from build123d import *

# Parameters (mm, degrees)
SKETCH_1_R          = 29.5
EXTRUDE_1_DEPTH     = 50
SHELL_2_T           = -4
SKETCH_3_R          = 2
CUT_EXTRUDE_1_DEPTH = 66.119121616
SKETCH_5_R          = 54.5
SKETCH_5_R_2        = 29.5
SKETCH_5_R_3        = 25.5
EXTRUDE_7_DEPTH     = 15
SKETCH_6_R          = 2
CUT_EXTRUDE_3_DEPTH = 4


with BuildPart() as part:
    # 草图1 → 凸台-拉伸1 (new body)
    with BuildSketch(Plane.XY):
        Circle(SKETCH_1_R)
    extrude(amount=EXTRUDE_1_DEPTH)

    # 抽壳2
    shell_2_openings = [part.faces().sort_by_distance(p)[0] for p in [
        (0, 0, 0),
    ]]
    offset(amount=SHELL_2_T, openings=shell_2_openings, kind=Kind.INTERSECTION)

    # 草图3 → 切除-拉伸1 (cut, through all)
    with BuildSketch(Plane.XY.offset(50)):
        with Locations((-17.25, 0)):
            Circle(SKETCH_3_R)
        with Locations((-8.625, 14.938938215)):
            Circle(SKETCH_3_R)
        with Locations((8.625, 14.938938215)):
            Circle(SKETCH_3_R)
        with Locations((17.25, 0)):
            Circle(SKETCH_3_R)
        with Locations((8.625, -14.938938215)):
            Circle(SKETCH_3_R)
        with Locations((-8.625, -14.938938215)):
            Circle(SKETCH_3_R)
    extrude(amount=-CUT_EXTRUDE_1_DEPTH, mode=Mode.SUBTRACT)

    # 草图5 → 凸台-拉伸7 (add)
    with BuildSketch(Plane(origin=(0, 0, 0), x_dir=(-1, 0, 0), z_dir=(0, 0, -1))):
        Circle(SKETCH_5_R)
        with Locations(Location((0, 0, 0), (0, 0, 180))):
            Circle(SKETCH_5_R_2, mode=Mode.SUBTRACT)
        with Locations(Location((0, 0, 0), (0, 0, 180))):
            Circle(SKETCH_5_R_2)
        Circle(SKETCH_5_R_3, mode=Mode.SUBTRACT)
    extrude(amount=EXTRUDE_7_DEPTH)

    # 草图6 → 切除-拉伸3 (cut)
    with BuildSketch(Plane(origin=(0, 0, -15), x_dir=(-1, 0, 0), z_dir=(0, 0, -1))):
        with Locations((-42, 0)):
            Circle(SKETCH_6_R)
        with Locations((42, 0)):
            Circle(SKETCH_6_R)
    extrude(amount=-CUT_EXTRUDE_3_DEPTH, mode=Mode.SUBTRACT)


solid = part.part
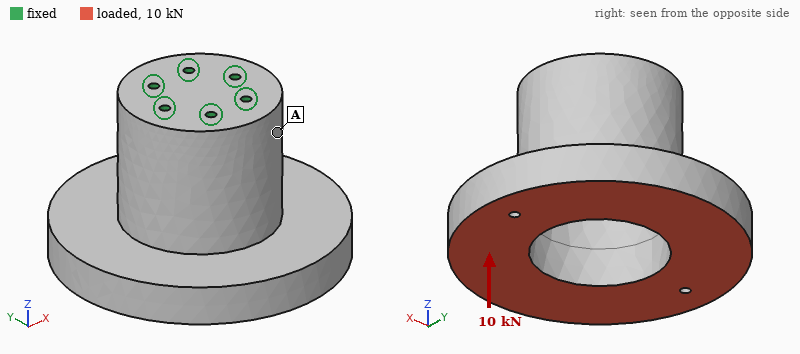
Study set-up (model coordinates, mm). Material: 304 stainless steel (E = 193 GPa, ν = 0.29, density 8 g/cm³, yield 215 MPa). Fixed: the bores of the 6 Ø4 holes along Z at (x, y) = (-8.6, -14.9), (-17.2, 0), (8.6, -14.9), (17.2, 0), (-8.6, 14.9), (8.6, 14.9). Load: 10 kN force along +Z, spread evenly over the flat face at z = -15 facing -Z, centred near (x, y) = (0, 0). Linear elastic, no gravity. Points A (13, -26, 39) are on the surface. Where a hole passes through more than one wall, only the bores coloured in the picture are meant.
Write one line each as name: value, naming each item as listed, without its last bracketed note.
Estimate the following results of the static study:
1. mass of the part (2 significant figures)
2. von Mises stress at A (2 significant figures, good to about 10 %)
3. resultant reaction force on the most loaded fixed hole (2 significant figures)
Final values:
mass of the part: 1.2 kg
von Mises stress at A: 20 MPa
resultant reaction force on the most loaded fixed hole: 1.7 kN
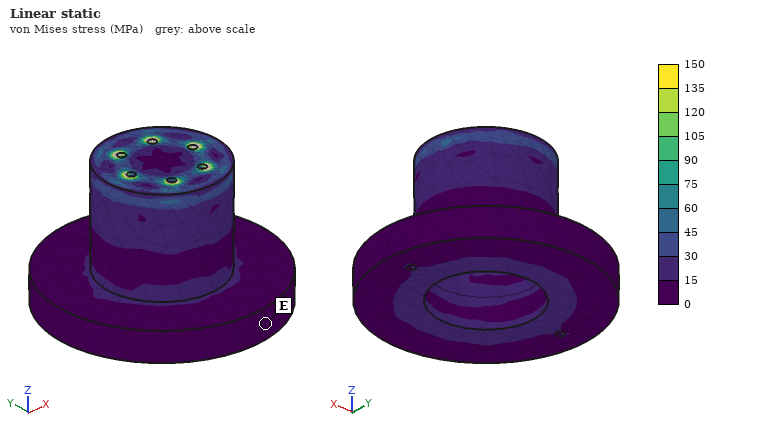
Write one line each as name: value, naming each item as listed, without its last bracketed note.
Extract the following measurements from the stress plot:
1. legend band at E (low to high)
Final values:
legend band at E: 0 to 15 MPa
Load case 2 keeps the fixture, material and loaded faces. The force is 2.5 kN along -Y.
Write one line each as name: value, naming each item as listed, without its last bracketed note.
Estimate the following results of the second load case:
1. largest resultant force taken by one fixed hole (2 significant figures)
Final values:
largest resultant force taken by one fixed hole: 2.0 kN
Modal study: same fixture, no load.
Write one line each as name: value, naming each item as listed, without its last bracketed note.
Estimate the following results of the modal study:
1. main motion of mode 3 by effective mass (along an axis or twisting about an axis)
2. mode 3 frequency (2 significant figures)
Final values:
main motion of mode 3 by effective mass: twisting about Z
mode 3 frequency: 2900 Hz
